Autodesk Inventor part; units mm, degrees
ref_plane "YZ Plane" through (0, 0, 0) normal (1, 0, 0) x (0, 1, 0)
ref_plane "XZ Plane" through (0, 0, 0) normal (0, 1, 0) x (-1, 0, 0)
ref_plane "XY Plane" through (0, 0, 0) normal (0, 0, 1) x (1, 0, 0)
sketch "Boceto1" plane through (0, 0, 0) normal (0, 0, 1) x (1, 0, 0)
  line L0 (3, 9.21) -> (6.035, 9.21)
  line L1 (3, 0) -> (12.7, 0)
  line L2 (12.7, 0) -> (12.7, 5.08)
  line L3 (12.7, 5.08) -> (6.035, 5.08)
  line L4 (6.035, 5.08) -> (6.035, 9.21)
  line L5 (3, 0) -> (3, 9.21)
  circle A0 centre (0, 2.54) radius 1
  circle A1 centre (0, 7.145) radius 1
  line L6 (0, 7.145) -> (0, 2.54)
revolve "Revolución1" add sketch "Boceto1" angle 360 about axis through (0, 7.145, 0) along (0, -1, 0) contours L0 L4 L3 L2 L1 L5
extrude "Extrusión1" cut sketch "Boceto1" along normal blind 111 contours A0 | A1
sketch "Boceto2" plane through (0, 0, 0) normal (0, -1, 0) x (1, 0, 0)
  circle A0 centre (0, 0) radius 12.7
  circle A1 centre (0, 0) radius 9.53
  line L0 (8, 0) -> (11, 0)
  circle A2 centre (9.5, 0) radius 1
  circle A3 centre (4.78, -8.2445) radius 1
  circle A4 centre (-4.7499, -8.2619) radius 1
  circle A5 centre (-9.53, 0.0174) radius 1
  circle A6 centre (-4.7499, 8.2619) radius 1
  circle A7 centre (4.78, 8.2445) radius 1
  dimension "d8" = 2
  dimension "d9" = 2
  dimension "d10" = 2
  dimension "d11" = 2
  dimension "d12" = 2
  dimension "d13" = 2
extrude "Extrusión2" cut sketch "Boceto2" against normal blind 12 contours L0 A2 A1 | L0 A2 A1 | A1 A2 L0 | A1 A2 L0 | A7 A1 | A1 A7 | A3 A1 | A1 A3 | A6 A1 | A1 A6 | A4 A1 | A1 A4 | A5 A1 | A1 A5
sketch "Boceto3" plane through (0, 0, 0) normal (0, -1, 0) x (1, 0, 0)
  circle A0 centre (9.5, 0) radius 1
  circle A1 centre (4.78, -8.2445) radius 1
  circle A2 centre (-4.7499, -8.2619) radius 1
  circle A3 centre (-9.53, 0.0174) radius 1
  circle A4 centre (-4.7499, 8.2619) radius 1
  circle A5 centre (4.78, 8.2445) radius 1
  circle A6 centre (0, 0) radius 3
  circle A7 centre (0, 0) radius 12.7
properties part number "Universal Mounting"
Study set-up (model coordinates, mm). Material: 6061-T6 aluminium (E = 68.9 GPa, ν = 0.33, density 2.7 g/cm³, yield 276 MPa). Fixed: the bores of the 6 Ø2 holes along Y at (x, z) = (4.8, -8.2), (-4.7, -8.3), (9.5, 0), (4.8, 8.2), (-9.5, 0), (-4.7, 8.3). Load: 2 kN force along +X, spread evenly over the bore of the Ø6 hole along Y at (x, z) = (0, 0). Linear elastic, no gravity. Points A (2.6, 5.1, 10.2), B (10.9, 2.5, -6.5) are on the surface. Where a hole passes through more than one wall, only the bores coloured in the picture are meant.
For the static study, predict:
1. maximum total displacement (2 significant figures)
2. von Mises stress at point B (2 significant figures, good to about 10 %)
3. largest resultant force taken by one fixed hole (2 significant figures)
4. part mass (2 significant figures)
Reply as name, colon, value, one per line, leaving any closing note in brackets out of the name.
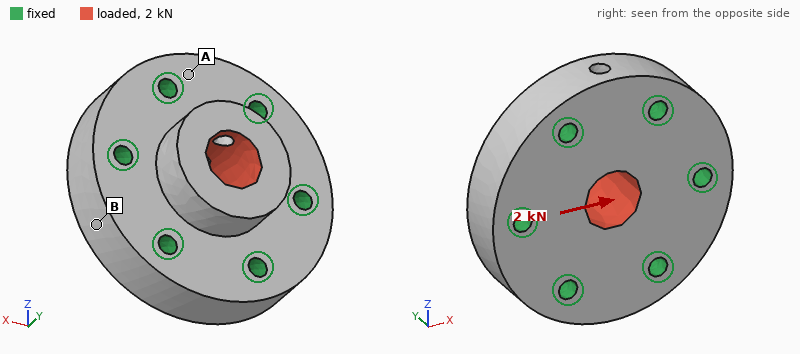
maximum total displacement: 4.7 µm
von Mises stress at point B: 6.1 MPa
largest resultant force taken by one fixed hole: 540 N
part mass: 7.2 g
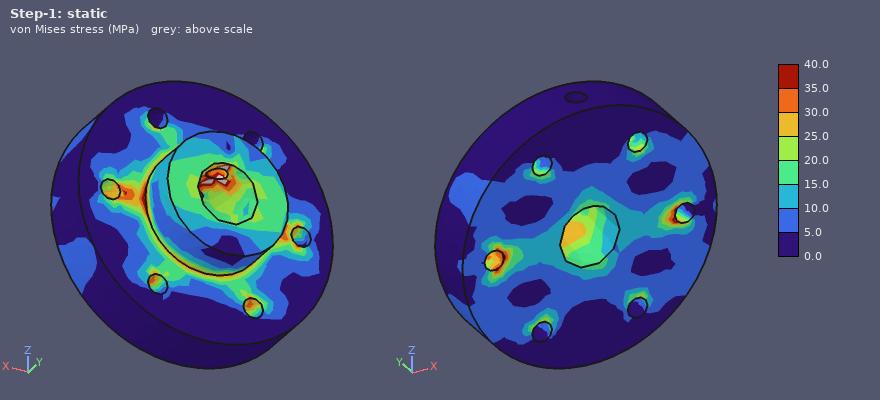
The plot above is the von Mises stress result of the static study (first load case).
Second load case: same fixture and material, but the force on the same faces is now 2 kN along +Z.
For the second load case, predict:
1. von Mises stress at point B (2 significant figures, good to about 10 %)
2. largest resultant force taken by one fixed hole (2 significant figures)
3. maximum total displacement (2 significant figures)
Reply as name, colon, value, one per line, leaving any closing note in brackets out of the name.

von Mises stress at point B: 3.4 MPa
largest resultant force taken by one fixed hole: 470 N
maximum total displacement: 4.4 µm
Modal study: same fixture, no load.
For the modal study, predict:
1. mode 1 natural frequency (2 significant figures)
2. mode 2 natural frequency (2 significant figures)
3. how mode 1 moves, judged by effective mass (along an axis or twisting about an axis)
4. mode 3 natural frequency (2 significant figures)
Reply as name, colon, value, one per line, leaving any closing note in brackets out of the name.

mode 1 natural frequency: 81 kHz
mode 2 natural frequency: 89 kHz
how mode 1 moves, judged by effective mass: along Y
mode 3 natural frequency: 90 kHz
